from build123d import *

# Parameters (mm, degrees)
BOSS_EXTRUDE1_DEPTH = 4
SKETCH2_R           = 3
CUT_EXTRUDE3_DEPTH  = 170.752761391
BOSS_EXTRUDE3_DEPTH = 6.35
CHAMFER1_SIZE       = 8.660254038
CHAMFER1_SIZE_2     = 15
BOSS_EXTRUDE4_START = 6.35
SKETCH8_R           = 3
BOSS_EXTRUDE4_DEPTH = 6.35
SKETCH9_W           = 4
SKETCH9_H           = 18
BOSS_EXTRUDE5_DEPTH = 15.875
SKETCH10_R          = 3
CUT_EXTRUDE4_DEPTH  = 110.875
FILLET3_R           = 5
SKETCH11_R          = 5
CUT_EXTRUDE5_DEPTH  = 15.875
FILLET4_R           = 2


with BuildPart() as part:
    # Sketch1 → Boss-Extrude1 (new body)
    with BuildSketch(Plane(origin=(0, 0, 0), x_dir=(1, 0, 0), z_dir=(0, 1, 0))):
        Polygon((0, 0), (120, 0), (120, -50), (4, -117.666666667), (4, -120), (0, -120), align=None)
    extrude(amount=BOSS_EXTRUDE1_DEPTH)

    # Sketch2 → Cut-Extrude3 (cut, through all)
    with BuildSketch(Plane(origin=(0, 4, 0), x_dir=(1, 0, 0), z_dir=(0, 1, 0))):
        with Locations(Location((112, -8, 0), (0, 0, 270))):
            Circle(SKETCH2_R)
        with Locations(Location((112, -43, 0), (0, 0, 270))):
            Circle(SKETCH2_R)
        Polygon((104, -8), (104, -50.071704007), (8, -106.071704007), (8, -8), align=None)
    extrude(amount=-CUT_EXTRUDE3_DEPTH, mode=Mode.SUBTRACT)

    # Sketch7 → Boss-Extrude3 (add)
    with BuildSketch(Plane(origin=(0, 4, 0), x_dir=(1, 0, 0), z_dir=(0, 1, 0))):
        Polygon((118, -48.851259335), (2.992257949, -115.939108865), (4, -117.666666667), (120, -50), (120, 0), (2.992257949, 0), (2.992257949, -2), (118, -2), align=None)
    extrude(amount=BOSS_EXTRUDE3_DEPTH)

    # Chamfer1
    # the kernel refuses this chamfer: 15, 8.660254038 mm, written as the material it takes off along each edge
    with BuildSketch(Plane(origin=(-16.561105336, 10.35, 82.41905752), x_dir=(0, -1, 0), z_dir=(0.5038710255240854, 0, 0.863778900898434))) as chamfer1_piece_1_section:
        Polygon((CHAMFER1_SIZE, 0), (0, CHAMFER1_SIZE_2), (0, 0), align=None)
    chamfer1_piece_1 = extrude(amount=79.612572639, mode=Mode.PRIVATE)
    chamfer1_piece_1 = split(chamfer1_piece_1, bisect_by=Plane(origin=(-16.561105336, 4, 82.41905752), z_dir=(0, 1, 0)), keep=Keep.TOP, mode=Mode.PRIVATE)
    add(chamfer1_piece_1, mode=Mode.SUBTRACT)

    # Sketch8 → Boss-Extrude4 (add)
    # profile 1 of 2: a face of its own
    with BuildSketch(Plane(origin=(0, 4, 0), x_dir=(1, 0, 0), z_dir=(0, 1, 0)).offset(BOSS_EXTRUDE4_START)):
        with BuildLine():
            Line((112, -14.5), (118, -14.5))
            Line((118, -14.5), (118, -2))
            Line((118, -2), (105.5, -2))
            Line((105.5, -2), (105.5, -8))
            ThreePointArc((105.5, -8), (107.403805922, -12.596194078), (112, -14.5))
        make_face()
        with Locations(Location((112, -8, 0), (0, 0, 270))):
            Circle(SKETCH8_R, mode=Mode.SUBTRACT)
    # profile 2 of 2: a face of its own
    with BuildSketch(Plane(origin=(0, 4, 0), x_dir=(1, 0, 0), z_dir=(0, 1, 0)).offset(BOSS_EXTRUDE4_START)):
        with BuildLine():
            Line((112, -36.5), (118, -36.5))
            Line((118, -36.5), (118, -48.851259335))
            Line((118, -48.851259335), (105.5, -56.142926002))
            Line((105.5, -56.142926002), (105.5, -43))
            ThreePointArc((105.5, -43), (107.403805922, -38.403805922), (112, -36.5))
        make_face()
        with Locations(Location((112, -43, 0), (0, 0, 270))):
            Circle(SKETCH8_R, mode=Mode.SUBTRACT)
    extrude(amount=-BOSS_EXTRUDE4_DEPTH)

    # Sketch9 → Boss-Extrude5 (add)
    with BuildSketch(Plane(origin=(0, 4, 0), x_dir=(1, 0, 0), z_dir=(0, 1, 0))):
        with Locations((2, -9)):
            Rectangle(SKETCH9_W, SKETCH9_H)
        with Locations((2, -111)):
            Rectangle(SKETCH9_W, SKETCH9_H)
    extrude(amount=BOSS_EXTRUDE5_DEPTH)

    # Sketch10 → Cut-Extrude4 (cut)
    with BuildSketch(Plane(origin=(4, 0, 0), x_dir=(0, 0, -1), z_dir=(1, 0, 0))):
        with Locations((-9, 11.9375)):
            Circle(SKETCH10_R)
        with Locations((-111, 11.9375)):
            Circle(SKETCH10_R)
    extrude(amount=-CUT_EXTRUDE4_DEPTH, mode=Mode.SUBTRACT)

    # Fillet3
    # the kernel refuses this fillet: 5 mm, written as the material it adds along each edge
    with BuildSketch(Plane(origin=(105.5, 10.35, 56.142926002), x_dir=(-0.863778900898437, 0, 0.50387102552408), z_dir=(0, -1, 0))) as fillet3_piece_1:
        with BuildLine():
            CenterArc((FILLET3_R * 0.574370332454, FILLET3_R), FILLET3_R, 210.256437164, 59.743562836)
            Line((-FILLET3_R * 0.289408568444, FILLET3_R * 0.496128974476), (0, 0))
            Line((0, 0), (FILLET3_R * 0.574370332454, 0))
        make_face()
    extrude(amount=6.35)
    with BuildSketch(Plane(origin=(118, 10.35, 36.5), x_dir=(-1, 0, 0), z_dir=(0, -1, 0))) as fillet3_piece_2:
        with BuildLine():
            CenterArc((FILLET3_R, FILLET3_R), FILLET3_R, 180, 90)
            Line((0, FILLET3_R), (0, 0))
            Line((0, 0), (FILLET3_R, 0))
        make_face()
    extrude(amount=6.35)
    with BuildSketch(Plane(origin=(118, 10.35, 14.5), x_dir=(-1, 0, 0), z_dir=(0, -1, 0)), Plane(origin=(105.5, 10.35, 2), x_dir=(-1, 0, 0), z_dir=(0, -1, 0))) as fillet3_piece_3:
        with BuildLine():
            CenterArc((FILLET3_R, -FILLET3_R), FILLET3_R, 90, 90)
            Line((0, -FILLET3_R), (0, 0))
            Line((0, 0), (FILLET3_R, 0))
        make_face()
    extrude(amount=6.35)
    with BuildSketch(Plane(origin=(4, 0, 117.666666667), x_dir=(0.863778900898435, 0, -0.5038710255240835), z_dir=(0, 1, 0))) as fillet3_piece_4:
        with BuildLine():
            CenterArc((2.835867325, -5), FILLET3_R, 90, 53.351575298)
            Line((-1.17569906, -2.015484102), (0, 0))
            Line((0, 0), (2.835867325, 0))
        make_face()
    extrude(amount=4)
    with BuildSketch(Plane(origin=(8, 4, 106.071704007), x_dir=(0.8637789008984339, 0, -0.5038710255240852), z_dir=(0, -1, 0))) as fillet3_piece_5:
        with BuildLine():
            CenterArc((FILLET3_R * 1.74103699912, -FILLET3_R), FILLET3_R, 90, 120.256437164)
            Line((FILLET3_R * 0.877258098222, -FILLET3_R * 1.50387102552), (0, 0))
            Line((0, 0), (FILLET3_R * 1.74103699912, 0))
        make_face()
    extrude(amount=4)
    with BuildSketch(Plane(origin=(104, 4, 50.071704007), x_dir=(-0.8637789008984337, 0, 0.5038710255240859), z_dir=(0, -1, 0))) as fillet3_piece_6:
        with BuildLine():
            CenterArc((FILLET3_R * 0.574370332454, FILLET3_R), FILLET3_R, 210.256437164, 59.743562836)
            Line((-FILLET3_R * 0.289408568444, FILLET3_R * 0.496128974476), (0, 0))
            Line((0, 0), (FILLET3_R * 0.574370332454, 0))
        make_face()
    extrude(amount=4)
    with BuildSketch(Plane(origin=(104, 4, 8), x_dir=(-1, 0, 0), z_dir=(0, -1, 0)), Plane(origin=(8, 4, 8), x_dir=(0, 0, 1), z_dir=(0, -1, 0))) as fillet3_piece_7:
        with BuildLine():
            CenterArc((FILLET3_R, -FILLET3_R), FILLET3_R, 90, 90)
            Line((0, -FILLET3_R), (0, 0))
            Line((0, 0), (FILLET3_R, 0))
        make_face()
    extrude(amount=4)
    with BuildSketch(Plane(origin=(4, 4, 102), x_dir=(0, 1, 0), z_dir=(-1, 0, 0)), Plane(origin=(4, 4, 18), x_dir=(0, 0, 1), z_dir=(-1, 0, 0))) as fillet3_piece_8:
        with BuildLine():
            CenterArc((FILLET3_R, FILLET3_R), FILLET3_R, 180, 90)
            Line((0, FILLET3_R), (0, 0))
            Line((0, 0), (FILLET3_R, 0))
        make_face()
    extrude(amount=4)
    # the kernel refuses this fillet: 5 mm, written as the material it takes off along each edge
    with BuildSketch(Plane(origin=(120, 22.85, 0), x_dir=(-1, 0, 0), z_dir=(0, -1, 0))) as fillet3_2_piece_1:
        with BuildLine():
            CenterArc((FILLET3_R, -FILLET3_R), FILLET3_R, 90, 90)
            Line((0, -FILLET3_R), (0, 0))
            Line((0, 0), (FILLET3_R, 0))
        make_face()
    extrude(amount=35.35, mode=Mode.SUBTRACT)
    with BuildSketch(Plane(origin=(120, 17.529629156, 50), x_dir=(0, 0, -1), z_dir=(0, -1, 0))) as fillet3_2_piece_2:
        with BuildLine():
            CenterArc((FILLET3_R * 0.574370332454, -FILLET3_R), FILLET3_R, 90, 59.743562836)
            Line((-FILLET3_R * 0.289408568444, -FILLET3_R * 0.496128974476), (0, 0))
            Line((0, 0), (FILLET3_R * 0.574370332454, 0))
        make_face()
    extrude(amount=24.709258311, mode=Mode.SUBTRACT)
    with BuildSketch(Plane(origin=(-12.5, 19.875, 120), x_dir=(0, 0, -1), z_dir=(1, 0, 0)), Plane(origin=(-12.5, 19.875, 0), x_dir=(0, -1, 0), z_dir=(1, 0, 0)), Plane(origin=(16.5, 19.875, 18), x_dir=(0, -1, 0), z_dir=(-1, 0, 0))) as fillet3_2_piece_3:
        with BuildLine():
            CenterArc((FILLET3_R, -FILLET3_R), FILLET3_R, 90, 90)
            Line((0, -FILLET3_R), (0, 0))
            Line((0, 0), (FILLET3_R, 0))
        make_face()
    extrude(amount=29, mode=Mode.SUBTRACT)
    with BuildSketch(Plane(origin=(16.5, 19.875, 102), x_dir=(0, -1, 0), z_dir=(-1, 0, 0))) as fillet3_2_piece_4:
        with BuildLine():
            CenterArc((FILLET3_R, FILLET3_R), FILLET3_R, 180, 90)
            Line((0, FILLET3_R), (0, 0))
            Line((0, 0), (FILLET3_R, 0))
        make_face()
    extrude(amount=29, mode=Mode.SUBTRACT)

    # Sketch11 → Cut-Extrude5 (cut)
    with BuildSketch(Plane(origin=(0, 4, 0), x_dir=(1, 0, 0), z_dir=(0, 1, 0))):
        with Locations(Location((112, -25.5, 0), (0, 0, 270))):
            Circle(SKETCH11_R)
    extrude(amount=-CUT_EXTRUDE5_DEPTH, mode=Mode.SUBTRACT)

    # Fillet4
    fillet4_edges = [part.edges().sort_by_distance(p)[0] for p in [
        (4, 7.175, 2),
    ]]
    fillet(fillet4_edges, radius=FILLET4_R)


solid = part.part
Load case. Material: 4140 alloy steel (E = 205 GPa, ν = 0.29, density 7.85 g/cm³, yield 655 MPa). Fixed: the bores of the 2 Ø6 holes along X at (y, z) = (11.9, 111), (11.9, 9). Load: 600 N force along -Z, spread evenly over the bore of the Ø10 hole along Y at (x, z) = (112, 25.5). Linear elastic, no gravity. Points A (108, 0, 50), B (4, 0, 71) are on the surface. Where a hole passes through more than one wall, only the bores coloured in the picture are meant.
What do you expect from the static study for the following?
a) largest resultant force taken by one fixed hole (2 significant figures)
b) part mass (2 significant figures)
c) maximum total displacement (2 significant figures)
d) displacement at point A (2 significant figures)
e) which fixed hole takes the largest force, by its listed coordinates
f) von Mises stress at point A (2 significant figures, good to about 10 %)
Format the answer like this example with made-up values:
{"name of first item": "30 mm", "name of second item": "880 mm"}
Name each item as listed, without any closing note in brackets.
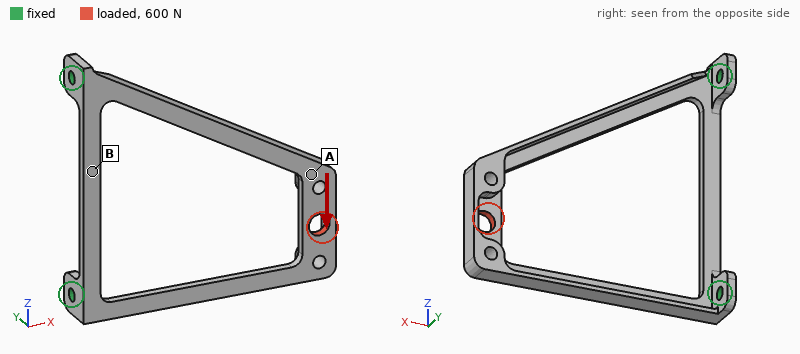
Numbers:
{"largest resultant force taken by one fixed hole": "640 N", "part mass": "160 g", "maximum total displacement": "0.40 mm", "displacement at point A": "0.33 mm", "which fixed hole takes the largest force, by its listed coordinates": "(11.9, 111)", "von Mises stress at point A": "50 MPa"}
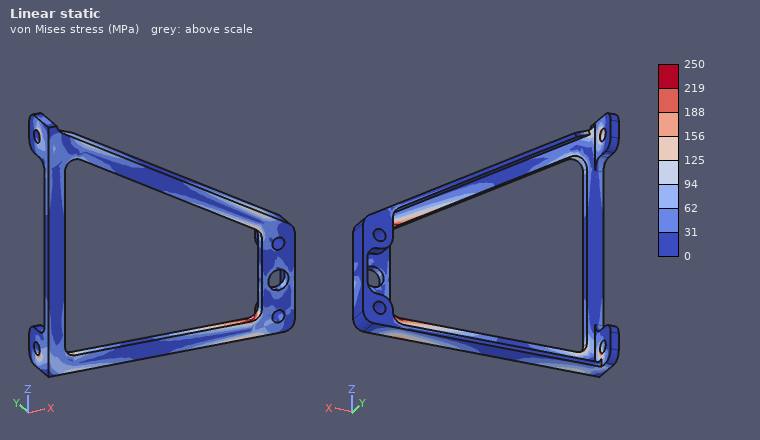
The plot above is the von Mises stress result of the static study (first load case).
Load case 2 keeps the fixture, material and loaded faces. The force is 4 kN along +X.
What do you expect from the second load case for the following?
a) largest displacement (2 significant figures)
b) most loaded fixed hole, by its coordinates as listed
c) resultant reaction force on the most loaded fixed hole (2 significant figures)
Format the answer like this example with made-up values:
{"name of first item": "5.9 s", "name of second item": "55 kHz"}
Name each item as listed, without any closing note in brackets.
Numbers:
{"largest displacement": "1.2 mm", "most loaded fixed hole, by its coordinates as listed": "(11.9, 9)", "resultant reaction force on the most loaded fixed hole": "3.1 kN"}
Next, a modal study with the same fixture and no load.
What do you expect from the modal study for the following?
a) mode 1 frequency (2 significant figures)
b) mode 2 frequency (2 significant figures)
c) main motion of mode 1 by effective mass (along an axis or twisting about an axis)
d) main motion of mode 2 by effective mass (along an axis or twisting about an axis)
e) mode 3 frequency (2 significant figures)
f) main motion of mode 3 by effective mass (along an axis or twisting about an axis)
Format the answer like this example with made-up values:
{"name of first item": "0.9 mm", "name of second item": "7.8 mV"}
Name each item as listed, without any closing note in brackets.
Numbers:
{"mode 1 frequency": "250 Hz", "mode 2 frequency": "640 Hz", "main motion of mode 1 by effective mass": "along Y", "main motion of mode 2 by effective mass": "along Z", "mode 3 frequency": "970 Hz", "main motion of mode 3 by effective mass": "along Z"}
